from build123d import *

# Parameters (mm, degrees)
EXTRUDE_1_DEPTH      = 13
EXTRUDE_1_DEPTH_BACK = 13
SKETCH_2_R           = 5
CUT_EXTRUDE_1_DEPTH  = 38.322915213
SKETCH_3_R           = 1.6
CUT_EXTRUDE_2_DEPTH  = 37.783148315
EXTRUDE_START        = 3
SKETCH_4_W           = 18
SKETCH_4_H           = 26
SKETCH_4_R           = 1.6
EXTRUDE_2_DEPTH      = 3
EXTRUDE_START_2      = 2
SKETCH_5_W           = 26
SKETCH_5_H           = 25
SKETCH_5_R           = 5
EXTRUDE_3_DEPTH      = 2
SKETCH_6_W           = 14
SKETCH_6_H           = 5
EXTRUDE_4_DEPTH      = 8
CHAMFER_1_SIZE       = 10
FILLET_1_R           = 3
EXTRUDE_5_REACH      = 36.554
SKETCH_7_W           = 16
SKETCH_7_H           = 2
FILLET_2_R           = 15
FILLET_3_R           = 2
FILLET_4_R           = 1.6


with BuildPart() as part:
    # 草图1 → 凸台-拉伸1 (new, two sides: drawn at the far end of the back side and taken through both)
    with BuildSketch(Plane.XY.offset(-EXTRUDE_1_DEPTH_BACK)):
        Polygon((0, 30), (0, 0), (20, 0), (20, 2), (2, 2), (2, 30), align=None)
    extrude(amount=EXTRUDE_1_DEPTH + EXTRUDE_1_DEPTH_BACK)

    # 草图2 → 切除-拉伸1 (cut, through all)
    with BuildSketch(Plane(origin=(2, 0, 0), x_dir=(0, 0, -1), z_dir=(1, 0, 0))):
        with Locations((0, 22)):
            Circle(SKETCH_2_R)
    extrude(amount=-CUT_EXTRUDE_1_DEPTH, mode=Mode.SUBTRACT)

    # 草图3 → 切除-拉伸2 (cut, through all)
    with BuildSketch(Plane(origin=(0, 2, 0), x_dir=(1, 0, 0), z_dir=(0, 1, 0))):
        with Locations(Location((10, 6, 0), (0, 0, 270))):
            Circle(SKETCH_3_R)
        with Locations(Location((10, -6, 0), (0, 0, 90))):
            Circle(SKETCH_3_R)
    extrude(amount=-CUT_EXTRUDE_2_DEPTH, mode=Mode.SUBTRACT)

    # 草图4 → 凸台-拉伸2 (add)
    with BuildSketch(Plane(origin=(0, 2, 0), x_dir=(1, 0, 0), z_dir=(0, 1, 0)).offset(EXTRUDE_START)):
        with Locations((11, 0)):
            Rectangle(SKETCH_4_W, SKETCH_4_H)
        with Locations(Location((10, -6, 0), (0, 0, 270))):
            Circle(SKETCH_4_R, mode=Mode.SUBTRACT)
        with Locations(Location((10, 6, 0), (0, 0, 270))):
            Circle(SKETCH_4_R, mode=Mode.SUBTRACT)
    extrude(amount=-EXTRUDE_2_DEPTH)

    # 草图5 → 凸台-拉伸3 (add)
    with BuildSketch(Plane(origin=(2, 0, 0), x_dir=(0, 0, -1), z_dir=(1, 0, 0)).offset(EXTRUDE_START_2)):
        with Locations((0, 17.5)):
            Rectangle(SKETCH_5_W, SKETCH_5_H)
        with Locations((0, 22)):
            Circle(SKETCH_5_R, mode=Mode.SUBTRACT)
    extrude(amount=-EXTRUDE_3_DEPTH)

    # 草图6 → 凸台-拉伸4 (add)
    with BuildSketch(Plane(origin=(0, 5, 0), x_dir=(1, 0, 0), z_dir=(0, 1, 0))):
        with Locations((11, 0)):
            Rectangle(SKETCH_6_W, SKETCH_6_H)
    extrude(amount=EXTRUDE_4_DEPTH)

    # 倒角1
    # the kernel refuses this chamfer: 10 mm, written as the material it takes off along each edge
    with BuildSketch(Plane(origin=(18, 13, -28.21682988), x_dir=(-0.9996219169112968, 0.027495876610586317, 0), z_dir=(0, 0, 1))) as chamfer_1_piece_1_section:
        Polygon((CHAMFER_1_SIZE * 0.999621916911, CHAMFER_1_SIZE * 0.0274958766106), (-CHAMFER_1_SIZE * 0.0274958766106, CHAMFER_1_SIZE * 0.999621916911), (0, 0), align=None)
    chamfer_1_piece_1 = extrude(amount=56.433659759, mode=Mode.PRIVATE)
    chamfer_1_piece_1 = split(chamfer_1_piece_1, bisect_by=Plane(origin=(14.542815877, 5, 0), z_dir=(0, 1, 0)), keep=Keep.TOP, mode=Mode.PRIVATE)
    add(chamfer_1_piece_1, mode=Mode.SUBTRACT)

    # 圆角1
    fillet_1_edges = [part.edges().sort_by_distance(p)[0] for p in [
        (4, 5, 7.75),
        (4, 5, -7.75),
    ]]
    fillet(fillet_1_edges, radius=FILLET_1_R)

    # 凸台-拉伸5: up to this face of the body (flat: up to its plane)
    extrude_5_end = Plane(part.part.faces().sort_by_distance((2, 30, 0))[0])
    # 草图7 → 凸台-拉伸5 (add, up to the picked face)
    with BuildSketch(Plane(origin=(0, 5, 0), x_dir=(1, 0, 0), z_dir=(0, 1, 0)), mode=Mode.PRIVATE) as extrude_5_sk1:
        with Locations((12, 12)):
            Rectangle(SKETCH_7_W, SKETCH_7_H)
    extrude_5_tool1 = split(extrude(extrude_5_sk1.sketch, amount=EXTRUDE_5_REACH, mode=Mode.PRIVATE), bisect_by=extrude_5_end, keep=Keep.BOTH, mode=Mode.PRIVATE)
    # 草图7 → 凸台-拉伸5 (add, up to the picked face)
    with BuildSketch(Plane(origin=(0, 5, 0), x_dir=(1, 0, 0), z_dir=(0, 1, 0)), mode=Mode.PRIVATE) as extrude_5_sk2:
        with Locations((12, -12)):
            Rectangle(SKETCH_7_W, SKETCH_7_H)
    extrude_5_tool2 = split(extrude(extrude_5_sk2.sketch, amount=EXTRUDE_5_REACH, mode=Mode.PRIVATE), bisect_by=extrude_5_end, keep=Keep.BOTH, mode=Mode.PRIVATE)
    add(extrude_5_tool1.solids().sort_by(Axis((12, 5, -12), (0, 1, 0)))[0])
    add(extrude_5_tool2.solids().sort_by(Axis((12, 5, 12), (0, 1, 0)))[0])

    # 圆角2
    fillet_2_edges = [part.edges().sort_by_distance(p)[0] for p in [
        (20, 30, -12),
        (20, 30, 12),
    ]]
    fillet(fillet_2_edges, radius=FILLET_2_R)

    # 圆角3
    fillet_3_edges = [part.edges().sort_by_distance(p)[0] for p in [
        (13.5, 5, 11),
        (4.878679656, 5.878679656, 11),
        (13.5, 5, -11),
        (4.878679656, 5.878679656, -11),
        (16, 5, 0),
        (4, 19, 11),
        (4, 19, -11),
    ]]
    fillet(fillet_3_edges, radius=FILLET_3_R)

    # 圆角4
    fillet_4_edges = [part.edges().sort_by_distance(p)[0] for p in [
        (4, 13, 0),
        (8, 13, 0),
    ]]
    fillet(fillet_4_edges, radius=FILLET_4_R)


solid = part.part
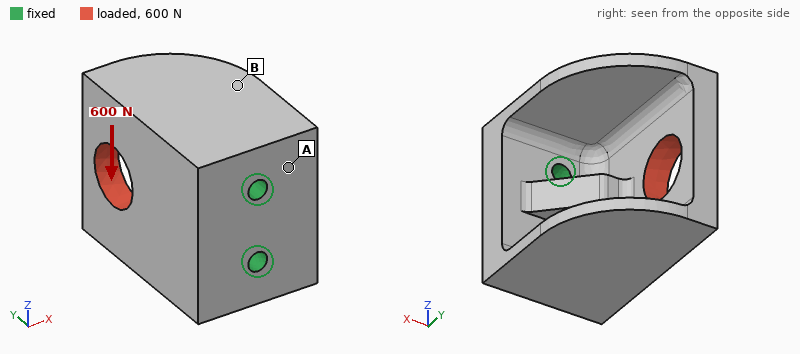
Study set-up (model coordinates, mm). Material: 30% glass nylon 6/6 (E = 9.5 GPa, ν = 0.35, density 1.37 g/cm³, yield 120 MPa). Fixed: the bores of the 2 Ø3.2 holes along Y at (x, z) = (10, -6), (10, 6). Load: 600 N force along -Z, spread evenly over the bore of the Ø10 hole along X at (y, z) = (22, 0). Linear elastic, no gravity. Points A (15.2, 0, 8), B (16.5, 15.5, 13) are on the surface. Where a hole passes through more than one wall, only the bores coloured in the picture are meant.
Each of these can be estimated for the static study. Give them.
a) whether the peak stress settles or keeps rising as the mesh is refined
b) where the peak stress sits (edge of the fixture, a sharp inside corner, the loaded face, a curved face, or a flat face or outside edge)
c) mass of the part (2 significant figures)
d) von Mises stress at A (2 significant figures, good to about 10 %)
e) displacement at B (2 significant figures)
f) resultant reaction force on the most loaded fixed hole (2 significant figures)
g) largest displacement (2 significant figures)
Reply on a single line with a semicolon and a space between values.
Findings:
keeps rising; edge of the fixture; 9.1 g; 14 MPa; 0.11 mm; 850 N; 0.29 mm
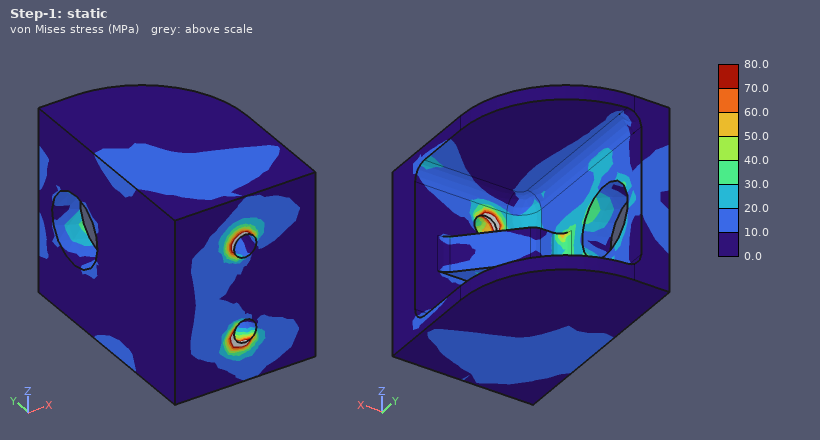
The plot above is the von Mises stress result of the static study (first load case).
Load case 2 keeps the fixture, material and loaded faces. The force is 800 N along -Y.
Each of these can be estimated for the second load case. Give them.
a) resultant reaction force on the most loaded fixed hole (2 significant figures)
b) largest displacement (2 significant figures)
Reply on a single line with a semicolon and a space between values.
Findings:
400 N; 0.19 mm
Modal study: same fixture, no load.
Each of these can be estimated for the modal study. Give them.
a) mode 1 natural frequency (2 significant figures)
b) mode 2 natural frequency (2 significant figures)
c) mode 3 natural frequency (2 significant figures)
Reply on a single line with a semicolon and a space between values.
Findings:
3800 Hz; 3900 Hz; 5800 Hz
